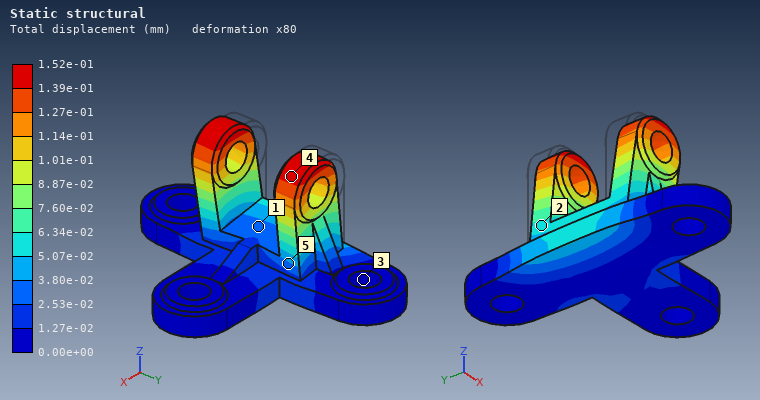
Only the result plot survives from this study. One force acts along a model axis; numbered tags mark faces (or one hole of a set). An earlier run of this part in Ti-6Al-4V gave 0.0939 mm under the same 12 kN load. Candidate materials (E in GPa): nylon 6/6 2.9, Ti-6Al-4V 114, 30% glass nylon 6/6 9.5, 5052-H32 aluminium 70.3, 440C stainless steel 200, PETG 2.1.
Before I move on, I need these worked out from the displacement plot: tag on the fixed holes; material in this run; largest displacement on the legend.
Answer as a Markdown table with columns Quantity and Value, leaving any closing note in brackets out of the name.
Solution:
| Quantity | Value |
|---|---|
| tag on the fixed holes | 3 |
| material in this run | 5052-H32 aluminium |
| largest displacement on the legend | 1.52e-01 mm |
